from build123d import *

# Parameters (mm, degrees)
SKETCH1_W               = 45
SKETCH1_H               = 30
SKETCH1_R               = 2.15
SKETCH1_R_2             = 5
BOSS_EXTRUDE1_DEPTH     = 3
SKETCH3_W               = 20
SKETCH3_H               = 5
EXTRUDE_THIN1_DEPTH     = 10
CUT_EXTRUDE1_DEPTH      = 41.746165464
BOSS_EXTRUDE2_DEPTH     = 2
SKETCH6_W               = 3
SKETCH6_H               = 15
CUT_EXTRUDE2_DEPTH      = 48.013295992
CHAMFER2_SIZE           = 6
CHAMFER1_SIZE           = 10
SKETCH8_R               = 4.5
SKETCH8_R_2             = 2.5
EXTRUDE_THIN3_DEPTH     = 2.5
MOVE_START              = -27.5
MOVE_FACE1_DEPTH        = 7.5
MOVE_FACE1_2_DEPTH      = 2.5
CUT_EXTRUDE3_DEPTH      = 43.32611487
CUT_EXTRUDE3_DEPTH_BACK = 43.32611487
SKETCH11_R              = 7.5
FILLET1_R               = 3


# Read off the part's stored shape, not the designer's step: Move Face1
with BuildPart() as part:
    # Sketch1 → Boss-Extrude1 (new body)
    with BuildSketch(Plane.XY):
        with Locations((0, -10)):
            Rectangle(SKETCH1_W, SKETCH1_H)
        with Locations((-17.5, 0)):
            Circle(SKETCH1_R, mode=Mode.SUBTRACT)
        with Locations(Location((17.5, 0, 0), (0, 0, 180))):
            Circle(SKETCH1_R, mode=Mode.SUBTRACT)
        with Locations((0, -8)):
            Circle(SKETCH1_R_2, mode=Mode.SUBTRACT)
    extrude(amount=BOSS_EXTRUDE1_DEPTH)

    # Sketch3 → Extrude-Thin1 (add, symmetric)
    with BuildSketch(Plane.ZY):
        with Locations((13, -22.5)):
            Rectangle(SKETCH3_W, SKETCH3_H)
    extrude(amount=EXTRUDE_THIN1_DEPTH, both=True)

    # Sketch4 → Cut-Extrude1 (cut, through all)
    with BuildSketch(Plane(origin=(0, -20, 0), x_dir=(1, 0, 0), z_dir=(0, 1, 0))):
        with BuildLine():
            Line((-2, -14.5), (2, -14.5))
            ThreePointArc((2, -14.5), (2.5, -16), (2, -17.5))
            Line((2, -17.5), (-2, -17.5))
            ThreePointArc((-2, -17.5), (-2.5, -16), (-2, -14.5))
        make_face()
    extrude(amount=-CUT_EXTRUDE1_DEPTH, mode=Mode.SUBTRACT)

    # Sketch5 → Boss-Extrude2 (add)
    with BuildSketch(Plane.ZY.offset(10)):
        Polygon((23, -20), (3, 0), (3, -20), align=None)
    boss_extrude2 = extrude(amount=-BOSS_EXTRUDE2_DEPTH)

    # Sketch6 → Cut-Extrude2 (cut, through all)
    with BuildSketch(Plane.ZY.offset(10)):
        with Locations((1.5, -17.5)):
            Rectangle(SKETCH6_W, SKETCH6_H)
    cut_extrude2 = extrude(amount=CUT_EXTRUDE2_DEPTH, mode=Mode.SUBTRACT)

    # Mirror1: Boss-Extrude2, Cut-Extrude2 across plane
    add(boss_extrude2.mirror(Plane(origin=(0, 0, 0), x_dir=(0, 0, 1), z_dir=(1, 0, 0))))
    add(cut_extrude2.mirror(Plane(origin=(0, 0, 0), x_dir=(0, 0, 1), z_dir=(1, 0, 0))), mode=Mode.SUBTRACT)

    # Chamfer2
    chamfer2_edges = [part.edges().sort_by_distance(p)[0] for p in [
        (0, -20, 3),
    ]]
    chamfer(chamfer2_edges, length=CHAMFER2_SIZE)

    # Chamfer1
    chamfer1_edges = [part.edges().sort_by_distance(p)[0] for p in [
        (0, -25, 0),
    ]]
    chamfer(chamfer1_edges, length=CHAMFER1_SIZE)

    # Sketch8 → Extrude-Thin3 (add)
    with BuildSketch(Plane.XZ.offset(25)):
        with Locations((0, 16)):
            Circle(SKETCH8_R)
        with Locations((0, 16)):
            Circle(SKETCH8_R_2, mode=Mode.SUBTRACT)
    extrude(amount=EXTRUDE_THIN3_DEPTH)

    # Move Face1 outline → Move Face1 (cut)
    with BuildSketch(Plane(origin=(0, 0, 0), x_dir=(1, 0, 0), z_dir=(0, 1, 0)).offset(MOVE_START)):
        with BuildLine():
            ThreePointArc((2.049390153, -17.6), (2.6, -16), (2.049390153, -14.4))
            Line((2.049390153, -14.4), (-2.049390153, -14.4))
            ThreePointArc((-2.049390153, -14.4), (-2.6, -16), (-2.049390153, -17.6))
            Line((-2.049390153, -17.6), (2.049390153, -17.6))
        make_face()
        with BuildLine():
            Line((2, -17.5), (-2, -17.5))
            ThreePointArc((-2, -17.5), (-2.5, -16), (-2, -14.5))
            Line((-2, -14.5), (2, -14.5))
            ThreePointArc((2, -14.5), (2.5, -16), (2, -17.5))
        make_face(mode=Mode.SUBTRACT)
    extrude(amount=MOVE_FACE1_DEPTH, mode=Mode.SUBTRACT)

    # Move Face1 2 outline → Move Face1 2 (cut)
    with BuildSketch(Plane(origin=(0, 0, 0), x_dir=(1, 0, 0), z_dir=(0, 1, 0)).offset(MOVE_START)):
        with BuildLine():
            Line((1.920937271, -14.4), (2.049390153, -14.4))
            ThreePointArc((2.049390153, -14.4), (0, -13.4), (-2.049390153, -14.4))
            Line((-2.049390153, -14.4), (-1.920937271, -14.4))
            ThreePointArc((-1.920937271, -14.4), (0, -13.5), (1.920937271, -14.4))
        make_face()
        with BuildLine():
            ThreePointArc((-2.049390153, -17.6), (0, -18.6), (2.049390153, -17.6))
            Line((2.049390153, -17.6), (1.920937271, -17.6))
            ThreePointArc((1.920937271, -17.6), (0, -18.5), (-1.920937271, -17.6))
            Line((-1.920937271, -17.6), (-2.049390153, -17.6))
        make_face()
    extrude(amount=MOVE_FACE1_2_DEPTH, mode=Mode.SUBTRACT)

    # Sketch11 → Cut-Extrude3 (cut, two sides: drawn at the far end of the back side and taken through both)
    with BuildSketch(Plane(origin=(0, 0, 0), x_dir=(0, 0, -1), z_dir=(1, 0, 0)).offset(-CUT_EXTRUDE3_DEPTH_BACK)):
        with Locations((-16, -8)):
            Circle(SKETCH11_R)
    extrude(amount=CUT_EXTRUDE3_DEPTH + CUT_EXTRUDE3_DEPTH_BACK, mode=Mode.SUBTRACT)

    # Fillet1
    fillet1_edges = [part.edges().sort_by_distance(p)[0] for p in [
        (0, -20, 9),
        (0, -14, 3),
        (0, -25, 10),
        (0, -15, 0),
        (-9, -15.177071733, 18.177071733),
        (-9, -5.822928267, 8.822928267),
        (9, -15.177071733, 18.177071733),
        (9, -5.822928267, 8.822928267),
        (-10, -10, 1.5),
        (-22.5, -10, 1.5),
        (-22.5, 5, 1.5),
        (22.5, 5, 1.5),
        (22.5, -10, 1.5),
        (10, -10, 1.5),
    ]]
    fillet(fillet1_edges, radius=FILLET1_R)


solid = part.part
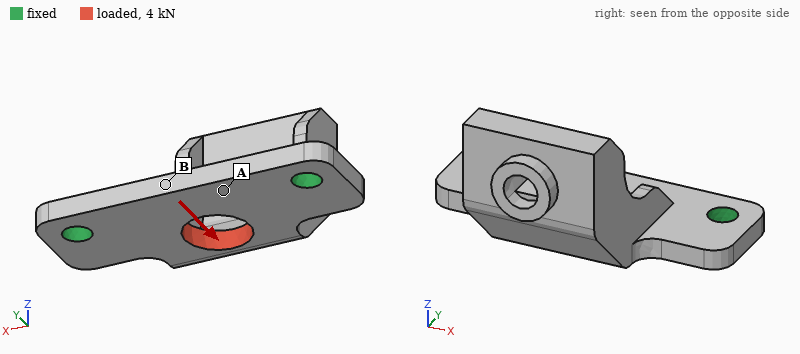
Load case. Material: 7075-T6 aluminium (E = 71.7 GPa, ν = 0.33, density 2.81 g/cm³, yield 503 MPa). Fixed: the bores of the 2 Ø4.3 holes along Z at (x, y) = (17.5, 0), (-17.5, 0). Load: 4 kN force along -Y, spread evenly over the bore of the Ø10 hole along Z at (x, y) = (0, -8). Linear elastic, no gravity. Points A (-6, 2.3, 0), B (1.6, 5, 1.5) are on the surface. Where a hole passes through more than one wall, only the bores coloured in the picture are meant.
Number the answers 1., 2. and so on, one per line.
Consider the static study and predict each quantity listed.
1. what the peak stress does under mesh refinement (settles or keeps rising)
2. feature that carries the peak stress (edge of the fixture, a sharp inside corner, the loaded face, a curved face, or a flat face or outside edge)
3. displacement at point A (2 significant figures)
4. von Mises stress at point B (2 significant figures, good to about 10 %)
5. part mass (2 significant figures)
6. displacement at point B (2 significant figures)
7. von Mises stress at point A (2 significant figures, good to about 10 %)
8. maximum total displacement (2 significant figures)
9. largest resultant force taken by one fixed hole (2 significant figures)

1. keeps rising
2. edge of the fixture
3. 30 µm
4. 110 MPa
5. 13 g
6. 37 µm
7. 45 MPa
8. 42 µm
9. 2.1 kN
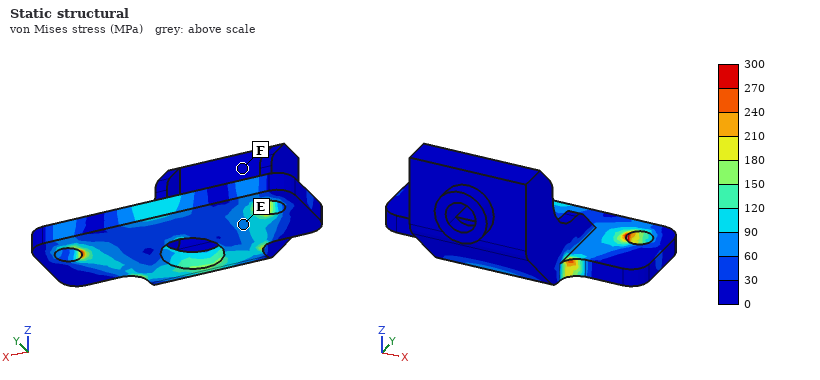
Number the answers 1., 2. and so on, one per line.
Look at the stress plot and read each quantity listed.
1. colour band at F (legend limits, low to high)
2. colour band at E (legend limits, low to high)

1. 0 to 30 MPa
2. 60 to 90 MPa
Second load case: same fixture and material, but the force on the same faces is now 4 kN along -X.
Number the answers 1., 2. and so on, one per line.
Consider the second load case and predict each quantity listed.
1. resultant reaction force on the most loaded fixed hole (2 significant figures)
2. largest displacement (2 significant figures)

1. 2.1 kN
2. 29 µm
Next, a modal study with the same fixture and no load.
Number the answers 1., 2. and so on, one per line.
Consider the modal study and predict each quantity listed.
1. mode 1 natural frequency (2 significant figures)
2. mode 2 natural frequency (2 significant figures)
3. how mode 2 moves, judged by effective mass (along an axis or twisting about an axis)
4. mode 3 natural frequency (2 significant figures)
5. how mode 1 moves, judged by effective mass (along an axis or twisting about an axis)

1. 2100 Hz
2. 4500 Hz
3. along X
4. 10 kHz
5. along Z
